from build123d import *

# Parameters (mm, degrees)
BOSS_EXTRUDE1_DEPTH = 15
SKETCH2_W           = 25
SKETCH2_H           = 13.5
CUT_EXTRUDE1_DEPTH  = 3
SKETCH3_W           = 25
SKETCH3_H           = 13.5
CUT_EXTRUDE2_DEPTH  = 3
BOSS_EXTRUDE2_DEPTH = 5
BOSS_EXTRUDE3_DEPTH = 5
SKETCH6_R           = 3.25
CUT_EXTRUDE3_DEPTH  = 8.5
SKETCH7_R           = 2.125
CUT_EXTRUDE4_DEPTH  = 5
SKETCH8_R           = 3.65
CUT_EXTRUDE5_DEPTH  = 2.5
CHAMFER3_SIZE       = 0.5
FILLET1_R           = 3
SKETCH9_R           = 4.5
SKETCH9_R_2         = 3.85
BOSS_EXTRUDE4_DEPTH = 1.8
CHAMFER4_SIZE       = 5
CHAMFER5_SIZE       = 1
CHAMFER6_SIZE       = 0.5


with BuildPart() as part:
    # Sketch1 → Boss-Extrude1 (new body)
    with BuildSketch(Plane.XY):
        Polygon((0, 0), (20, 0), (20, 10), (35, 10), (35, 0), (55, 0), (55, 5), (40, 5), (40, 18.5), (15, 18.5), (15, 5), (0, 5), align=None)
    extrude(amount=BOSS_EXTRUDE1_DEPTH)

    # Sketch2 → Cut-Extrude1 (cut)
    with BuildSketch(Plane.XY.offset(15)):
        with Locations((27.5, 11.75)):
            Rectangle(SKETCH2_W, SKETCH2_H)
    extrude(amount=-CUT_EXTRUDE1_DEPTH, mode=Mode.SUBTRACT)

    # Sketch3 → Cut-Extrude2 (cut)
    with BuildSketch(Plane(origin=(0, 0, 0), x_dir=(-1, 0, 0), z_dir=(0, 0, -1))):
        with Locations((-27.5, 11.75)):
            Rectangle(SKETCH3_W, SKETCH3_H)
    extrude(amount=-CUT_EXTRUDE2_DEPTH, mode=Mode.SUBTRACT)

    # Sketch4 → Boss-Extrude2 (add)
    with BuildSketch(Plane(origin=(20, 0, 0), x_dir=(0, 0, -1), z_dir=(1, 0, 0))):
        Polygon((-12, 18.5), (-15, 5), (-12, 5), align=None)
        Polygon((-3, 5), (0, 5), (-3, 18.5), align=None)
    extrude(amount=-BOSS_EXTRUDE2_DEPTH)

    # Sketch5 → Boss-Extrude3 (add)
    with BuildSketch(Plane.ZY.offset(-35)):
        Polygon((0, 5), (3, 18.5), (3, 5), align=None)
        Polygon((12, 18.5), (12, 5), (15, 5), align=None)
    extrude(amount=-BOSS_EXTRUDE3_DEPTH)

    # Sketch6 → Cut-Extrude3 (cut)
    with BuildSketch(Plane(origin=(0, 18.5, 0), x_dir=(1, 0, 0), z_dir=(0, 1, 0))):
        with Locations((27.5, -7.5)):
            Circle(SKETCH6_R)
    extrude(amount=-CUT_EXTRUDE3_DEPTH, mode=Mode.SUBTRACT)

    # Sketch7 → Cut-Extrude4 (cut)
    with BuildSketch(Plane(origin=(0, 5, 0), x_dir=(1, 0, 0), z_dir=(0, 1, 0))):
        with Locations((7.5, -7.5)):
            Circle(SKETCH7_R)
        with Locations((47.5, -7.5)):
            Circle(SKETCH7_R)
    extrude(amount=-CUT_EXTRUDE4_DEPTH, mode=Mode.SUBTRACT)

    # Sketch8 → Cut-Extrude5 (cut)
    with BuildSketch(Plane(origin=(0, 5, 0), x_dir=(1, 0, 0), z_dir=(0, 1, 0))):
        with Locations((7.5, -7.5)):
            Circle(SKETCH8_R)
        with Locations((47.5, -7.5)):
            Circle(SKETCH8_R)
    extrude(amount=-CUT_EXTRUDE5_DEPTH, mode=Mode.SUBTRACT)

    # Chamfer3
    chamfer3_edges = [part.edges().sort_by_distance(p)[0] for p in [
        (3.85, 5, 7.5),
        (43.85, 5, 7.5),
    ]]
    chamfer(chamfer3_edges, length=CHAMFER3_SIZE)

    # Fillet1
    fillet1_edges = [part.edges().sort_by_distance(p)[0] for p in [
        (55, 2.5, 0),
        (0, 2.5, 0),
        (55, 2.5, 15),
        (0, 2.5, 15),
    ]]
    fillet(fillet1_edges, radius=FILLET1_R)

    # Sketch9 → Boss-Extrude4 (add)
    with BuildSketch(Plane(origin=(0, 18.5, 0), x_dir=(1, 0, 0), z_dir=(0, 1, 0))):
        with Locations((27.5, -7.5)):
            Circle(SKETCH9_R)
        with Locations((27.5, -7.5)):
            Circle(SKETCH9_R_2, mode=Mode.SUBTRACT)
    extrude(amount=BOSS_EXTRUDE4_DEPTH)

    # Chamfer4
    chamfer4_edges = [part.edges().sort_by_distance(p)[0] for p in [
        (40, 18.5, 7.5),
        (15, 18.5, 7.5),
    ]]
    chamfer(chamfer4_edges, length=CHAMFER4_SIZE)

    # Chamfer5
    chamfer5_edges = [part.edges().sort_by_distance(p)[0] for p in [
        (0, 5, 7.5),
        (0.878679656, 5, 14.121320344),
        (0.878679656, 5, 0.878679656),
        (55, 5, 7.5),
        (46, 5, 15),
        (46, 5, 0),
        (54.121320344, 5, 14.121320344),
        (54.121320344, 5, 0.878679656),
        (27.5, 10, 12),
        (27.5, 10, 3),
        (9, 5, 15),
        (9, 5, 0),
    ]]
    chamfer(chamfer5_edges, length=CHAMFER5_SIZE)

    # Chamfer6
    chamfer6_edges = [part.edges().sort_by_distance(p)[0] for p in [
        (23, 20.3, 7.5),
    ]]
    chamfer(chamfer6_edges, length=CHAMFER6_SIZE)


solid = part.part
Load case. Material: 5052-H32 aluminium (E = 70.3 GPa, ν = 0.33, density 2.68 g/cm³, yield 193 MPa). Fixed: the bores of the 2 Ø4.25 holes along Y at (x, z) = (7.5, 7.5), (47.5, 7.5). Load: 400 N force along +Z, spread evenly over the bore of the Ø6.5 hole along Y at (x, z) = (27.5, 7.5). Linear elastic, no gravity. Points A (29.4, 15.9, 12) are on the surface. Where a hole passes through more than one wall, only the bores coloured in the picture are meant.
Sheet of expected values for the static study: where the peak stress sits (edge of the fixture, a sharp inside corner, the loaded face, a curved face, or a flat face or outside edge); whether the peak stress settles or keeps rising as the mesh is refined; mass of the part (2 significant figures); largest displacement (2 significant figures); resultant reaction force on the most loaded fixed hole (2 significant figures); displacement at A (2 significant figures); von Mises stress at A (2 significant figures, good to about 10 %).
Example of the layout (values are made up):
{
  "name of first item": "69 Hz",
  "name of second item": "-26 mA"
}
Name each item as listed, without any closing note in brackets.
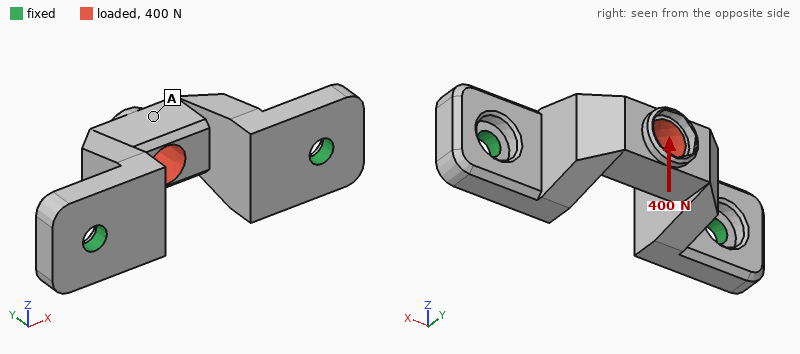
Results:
{
  "where the peak stress sits": "edge of the fixture",
  "whether the peak stress settles or keeps rising as the mesh is refined": "keeps rising",
  "mass of the part": "13 g",
  "largest displacement": "58 µm",
  "resultant reaction force on the most loaded fixed hole": "200 N",
  "displacement at A": "47 µm",
  "von Mises stress at A": "15 MPa"
}
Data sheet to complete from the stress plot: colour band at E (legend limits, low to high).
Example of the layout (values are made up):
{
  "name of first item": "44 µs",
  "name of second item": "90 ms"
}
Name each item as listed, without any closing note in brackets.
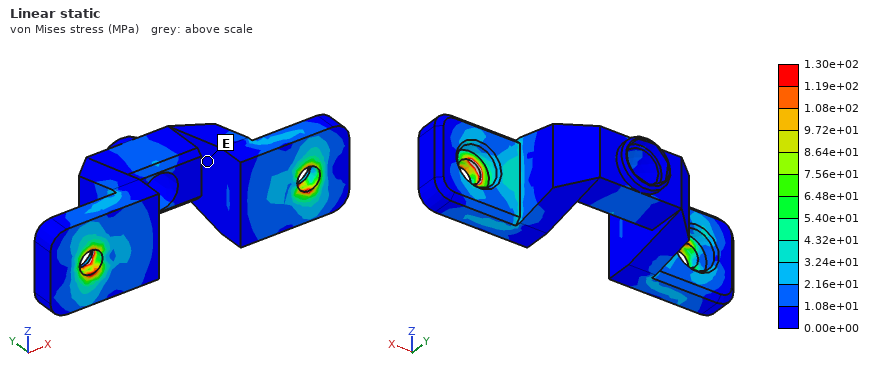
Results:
{
  "colour band at E": "0.00e+00 to 1.08e+01 MPa"
}
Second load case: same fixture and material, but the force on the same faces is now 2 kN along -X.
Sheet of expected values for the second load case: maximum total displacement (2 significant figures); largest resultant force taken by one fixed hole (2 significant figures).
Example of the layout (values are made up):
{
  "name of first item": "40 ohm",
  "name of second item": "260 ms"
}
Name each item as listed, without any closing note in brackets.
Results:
{
  "maximum total displacement": "28 µm",
  "largest resultant force taken by one fixed hole": "1.2 kN"
}
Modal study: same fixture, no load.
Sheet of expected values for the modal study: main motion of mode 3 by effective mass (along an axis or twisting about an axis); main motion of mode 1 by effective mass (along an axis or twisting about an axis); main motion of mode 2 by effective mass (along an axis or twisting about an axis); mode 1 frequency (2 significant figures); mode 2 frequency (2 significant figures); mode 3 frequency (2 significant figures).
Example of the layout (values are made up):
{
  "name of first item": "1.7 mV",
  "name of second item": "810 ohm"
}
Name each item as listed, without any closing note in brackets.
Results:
{
  "main motion of mode 3 by effective mass": "along X",
  "main motion of mode 1 by effective mass": "along Z",
  "main motion of mode 2 by effective mass": "along Y",
  "mode 1 frequency": "6900 Hz",
  "mode 2 frequency": "16 kHz",
  "mode 3 frequency": "17 kHz"
}
